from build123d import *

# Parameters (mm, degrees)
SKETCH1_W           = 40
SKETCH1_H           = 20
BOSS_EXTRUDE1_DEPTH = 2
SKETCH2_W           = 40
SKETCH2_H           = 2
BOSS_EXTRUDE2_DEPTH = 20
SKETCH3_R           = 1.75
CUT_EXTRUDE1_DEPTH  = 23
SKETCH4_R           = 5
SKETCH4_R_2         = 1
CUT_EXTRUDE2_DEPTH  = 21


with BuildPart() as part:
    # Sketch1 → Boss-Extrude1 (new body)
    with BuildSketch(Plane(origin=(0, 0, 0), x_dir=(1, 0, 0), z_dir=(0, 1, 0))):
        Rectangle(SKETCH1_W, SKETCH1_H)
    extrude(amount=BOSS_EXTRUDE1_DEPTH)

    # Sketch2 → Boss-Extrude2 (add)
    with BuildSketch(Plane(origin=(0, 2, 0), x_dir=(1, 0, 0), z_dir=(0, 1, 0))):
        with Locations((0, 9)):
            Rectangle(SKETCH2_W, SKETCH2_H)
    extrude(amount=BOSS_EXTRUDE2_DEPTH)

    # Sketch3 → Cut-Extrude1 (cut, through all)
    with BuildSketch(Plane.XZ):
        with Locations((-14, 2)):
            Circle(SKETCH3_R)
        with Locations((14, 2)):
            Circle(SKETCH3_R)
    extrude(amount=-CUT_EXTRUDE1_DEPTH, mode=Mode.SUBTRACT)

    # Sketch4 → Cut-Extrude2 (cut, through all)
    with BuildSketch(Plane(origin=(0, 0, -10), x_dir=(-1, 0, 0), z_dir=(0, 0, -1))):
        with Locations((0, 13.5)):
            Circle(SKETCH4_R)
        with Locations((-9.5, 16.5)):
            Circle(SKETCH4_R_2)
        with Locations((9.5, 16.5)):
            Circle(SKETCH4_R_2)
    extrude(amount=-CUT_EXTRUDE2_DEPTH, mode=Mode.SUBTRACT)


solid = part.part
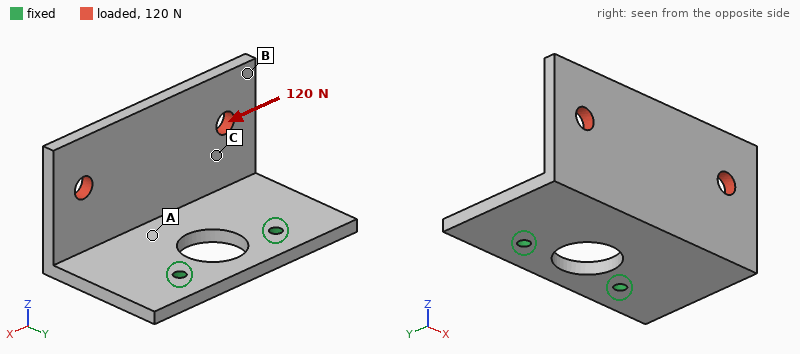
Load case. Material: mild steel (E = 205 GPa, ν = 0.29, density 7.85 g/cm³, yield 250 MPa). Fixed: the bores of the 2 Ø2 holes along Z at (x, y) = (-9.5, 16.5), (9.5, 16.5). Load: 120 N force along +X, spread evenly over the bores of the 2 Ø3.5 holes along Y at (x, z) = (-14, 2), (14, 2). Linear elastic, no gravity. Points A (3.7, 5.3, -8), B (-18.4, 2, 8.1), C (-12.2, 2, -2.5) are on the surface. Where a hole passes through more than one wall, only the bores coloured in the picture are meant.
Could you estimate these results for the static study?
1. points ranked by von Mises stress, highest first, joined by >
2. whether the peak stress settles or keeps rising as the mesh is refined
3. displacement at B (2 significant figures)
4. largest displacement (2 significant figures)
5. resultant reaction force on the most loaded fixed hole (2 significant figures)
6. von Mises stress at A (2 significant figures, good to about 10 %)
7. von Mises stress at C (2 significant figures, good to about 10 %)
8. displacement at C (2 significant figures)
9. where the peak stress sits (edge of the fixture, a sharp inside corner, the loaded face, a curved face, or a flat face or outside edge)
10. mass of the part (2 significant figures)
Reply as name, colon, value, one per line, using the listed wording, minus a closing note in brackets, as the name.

points ranked by von Mises stress, highest first, joined by >: A > C > B
whether the peak stress settles or keeps rising as the mesh is refined: keeps rising
displacement at B: 31 µm
largest displacement: 34 µm
resultant reaction force on the most loaded fixed hole: 110 N
von Mises stress at A: 31 MPa
von Mises stress at C: 16 MPa
displacement at C: 17 µm
where the peak stress sits: edge of the fixture
mass of the part: 23 g
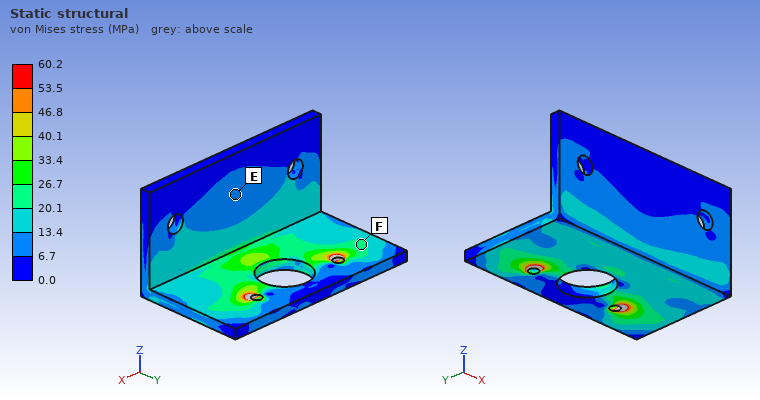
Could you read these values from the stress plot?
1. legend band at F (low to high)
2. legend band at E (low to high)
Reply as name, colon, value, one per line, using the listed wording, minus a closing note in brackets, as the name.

legend band at F: 20.1 to 26.7 MPa
legend band at E: 6.7 to 13.4 MPa
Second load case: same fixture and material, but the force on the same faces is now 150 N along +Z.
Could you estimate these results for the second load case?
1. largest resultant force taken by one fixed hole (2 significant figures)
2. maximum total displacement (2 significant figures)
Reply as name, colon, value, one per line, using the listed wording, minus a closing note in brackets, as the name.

largest resultant force taken by one fixed hole: 75 N
maximum total displacement: 0.10 mm
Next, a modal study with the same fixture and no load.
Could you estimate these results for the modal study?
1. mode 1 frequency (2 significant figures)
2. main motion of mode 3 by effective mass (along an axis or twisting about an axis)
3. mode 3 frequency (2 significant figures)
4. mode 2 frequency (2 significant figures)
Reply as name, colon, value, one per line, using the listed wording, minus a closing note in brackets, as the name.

mode 1 frequency: 1600 Hz
main motion of mode 3 by effective mass: along Z
mode 3 frequency: 4800 Hz
mode 2 frequency: 2800 Hz
